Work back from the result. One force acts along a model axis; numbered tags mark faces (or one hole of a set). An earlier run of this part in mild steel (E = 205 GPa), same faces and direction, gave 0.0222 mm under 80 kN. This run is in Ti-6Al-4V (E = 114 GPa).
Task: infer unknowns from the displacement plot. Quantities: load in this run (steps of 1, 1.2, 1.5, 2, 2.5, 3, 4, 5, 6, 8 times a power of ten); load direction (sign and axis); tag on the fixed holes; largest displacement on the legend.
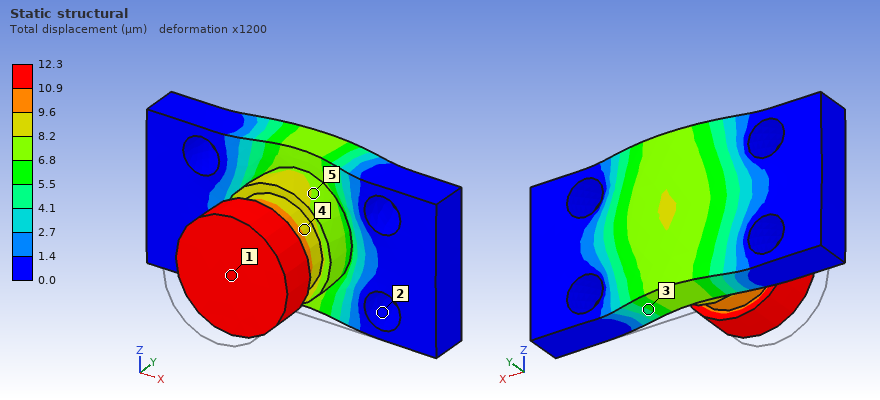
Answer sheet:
25 kN
+Y
2
12.3 µm
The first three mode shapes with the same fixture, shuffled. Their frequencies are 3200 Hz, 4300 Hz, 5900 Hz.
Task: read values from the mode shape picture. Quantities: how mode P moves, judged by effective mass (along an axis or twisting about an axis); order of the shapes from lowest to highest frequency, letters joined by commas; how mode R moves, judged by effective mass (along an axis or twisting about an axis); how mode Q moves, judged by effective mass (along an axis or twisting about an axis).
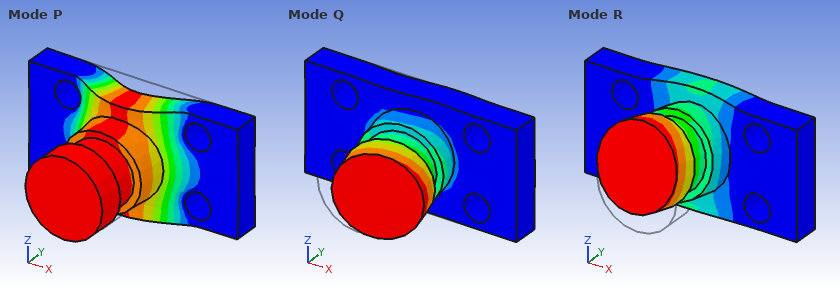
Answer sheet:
along Y
R, Q, P
along Z
along X
